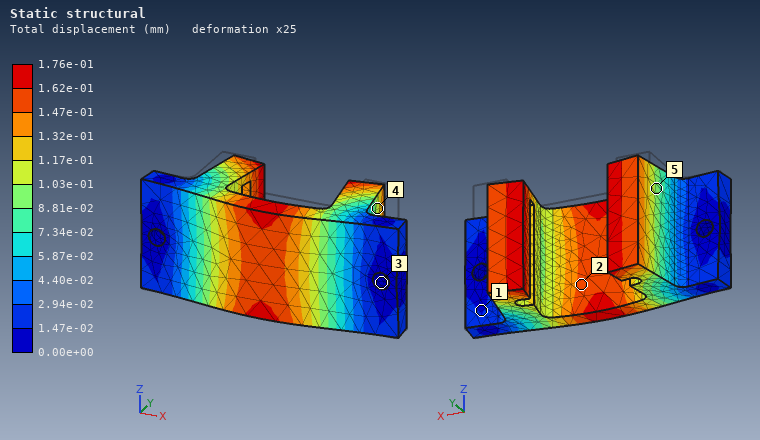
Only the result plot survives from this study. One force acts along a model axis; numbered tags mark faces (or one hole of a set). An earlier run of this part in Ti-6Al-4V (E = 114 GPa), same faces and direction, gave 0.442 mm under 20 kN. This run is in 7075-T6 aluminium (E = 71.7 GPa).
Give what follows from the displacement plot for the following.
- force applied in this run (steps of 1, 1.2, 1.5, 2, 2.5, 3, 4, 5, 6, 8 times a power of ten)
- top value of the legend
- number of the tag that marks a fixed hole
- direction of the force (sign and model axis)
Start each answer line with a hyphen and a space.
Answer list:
- 5 kN
- 1.76e-01 mm
- 3
- -Y
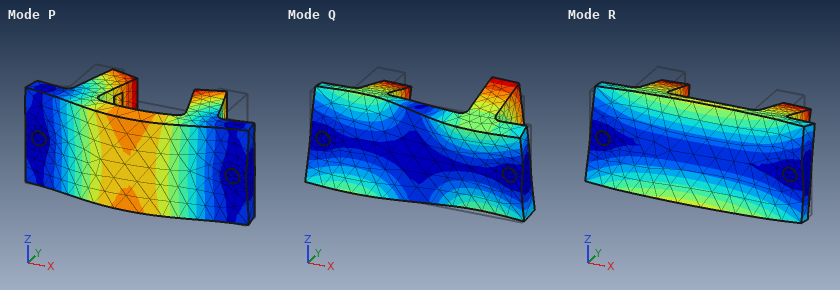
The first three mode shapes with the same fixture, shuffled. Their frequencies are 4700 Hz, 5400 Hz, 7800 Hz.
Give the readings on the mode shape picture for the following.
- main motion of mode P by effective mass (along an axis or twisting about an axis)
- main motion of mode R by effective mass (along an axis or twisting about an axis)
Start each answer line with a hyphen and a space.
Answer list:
- along Y
- along Z
